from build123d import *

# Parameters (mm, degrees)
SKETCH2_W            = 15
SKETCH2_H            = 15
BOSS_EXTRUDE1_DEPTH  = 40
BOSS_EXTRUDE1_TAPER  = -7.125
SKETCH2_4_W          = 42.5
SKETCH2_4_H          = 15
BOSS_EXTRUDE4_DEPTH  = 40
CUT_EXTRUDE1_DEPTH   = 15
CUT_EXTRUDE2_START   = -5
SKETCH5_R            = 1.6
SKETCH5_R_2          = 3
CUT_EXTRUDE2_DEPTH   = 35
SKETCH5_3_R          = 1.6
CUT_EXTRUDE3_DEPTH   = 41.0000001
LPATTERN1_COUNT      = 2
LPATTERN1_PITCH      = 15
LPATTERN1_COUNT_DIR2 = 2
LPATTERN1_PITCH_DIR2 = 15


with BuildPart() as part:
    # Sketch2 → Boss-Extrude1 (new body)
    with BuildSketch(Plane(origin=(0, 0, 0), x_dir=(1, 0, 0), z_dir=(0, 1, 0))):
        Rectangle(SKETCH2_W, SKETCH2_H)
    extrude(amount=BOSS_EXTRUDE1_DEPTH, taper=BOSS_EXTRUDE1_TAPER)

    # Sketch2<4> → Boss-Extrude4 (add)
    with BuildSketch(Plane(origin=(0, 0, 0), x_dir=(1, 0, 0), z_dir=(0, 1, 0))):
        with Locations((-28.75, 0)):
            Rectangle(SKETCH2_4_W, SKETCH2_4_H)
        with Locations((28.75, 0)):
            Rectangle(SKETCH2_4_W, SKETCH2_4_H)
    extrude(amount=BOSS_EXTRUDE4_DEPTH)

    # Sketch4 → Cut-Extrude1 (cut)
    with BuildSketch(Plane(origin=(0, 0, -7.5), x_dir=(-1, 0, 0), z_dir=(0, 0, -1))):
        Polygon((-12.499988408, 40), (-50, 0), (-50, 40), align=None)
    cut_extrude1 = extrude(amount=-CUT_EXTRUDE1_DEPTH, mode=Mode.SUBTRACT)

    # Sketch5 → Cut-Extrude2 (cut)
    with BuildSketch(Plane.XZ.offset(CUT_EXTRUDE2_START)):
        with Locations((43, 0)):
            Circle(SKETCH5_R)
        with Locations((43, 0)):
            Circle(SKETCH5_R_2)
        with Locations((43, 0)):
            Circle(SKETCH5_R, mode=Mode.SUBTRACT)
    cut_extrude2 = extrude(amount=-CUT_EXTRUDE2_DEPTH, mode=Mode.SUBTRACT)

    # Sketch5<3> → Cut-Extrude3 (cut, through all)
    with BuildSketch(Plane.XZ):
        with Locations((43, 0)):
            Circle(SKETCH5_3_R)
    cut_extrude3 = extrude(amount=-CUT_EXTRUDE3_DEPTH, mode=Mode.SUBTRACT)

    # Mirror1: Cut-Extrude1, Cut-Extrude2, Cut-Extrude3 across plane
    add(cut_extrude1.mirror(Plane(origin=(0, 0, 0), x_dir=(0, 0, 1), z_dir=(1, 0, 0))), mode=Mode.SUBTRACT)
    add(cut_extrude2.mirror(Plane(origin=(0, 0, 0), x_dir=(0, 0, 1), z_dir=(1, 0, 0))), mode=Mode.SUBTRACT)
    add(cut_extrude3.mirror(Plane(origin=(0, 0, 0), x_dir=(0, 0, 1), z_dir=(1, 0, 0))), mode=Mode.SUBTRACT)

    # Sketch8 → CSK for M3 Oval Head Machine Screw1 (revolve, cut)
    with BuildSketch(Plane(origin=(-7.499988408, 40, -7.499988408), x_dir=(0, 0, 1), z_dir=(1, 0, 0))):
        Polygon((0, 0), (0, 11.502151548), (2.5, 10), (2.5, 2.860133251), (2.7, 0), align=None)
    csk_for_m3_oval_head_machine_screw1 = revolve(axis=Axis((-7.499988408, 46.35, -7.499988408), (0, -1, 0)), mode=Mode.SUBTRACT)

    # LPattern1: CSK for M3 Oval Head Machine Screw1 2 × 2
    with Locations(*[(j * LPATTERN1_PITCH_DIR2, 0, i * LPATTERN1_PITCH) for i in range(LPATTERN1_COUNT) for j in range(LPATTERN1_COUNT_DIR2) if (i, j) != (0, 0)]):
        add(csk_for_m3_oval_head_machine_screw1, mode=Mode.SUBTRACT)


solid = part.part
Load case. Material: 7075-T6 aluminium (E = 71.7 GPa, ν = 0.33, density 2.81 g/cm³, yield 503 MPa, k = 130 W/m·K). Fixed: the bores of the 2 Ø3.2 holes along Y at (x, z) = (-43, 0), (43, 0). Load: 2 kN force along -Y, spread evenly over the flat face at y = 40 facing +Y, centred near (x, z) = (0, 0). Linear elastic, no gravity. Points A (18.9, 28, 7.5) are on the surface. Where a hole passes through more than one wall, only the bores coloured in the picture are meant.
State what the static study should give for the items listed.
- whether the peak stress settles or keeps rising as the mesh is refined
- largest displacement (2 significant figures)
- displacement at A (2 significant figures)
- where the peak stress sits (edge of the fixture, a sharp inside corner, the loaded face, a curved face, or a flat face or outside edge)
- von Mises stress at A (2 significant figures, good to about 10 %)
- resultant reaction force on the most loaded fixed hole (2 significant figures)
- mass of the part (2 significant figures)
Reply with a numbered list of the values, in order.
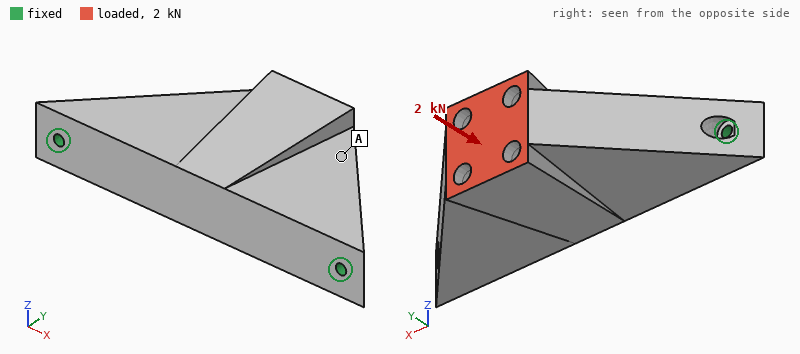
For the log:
1. keeps rising
2. 11 µm
3. 8.9 µm
4. edge of the fixture
5. 6.3 MPa
6. 1.3 kN
7. 110 g
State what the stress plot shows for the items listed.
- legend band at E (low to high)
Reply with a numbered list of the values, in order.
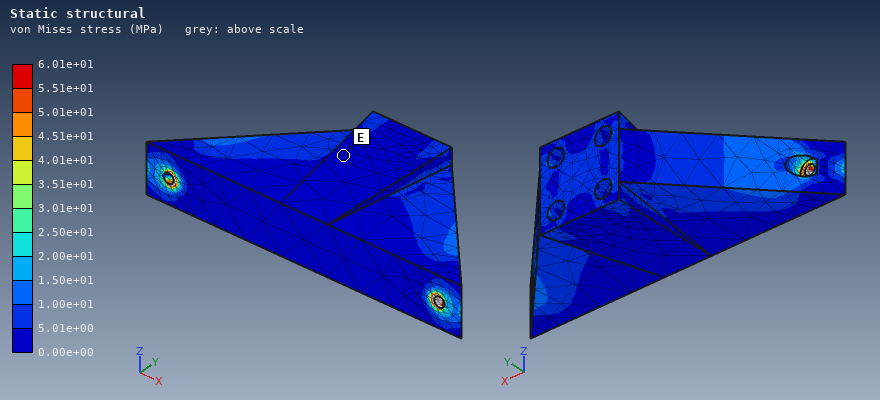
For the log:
1. 0.00e+00 to 5.01e+00 MPa
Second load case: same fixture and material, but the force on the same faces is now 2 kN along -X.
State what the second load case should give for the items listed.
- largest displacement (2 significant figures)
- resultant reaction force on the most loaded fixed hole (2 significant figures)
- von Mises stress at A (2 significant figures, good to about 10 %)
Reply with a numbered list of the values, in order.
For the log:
1. 11 µm
2. 1.3 kN
3. 6.4 MPa
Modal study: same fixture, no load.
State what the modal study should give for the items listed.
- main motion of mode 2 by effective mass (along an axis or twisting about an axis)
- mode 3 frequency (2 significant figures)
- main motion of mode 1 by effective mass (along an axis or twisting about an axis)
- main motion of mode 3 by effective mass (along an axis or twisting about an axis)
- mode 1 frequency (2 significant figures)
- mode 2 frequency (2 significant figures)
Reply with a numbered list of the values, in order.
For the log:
1. along Z
2. 7400 Hz
3. along Z
4. along Y
5. 1900 Hz
6. 7000 Hz
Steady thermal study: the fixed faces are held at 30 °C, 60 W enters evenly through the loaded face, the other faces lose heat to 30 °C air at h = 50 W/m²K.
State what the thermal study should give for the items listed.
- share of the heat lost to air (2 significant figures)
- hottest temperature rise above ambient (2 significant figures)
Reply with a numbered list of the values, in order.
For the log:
1. 21 %
2. 47 K
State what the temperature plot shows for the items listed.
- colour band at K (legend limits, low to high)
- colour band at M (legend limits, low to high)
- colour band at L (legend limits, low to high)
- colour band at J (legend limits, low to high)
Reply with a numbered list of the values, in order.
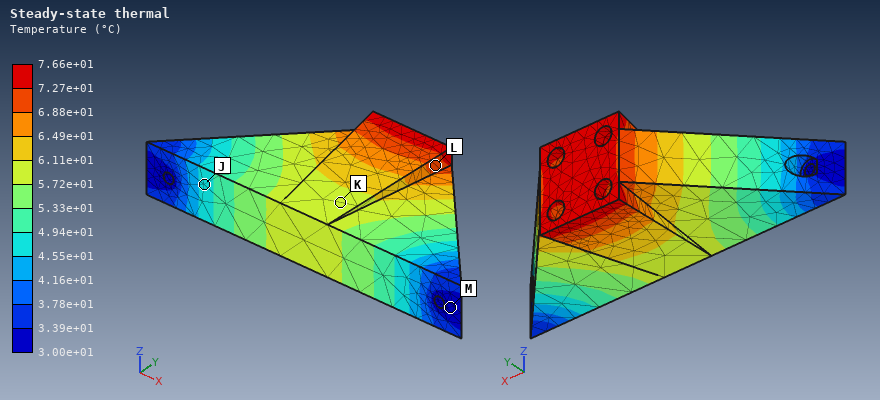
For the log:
1. 5.72e+01 to 6.11e+01 °C
2. 3.00e+01 to 3.39e+01 °C
3. 6.88e+01 to 7.27e+01 °C
4. 4.55e+01 to 4.94e+01 °C
